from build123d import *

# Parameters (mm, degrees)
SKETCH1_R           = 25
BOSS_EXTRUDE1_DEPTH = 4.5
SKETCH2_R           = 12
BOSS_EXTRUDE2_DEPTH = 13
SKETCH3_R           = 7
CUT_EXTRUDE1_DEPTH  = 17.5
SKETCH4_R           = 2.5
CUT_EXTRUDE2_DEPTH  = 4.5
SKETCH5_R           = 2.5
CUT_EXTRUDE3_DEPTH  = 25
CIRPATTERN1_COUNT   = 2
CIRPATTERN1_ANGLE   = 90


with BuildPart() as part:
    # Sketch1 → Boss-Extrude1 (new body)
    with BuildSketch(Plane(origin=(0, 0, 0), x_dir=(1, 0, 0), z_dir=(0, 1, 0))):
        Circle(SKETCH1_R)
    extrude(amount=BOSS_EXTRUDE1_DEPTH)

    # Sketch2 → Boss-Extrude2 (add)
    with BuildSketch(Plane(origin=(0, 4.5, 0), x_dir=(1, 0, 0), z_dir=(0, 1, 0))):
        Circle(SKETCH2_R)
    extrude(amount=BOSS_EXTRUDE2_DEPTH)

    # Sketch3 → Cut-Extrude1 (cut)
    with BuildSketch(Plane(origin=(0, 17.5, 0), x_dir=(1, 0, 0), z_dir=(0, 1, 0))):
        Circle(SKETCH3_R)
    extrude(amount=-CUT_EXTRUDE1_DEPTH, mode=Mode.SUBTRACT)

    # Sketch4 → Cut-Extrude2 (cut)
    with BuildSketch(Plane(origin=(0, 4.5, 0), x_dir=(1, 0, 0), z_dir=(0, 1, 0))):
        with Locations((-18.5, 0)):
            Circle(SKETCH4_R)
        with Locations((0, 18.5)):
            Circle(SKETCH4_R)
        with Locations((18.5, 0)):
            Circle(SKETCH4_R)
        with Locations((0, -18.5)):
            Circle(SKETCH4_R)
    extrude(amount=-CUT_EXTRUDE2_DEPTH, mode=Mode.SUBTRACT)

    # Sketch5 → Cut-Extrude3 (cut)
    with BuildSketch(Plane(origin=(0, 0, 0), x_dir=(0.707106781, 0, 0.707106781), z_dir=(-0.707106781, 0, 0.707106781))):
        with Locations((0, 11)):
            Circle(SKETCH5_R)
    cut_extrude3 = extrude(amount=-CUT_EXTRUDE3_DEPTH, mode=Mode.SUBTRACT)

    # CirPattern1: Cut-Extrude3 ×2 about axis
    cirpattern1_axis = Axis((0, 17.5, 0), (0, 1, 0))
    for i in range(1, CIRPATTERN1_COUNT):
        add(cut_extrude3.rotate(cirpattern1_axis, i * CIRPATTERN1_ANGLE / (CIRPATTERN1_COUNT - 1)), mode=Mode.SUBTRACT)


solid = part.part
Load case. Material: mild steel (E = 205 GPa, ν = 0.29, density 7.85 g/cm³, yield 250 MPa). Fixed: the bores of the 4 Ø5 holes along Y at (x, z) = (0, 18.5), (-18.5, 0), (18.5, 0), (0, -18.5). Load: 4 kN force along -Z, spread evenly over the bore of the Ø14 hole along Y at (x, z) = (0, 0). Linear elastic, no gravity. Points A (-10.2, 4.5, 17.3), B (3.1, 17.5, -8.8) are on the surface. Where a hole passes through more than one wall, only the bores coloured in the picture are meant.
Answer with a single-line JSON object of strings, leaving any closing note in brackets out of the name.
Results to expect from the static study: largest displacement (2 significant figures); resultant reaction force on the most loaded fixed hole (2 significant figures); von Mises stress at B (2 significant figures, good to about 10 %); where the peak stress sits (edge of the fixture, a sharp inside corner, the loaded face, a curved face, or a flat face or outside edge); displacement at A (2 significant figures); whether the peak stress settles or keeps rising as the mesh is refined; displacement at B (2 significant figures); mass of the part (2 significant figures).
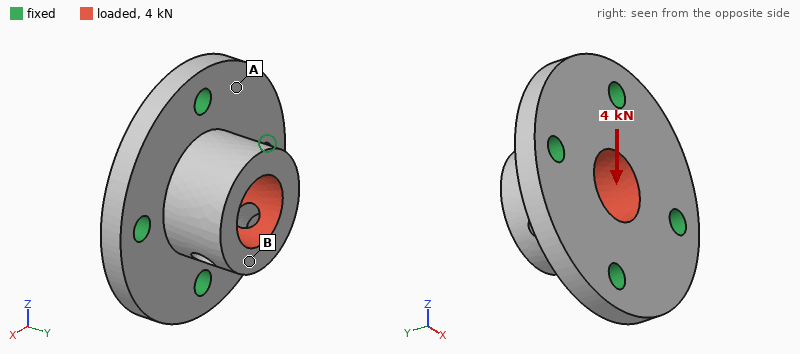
{"largest displacement": "5.9 µm", "resultant reaction force on the most loaded fixed hole": "1.5 kN", "von Mises stress at B": "17 MPa", "where the peak stress sits": "edge of the fixture", "displacement at A": "0.90 µm", "whether the peak stress settles or keeps rising as the mesh is refined": "keeps rising", "displacement at B": "5.5 µm", "mass of the part": "90 g"}
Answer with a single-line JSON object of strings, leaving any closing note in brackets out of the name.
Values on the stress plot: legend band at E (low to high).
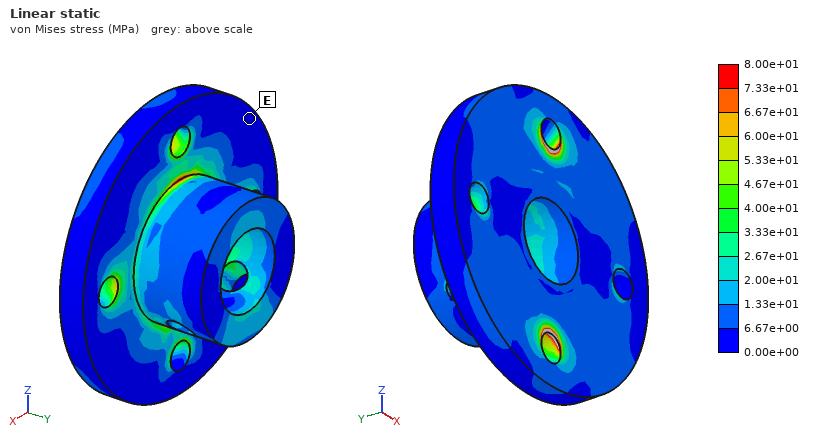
{"legend band at E": "0.00e+00 to 6.67e+00 MPa"}
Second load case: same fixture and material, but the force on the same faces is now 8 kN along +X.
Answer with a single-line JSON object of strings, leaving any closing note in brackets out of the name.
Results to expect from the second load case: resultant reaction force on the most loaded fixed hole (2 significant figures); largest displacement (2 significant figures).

{"resultant reaction force on the most loaded fixed hole": "2.9 kN", "largest displacement": "12 µm"}
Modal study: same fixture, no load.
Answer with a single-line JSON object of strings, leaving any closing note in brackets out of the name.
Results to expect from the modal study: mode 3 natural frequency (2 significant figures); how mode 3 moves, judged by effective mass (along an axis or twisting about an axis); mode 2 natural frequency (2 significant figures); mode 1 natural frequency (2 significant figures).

{"mode 3 natural frequency": "24 kHz", "how mode 3 moves, judged by effective mass": "along Y", "mode 2 natural frequency": "22 kHz", "mode 1 natural frequency": "22 kHz"}
